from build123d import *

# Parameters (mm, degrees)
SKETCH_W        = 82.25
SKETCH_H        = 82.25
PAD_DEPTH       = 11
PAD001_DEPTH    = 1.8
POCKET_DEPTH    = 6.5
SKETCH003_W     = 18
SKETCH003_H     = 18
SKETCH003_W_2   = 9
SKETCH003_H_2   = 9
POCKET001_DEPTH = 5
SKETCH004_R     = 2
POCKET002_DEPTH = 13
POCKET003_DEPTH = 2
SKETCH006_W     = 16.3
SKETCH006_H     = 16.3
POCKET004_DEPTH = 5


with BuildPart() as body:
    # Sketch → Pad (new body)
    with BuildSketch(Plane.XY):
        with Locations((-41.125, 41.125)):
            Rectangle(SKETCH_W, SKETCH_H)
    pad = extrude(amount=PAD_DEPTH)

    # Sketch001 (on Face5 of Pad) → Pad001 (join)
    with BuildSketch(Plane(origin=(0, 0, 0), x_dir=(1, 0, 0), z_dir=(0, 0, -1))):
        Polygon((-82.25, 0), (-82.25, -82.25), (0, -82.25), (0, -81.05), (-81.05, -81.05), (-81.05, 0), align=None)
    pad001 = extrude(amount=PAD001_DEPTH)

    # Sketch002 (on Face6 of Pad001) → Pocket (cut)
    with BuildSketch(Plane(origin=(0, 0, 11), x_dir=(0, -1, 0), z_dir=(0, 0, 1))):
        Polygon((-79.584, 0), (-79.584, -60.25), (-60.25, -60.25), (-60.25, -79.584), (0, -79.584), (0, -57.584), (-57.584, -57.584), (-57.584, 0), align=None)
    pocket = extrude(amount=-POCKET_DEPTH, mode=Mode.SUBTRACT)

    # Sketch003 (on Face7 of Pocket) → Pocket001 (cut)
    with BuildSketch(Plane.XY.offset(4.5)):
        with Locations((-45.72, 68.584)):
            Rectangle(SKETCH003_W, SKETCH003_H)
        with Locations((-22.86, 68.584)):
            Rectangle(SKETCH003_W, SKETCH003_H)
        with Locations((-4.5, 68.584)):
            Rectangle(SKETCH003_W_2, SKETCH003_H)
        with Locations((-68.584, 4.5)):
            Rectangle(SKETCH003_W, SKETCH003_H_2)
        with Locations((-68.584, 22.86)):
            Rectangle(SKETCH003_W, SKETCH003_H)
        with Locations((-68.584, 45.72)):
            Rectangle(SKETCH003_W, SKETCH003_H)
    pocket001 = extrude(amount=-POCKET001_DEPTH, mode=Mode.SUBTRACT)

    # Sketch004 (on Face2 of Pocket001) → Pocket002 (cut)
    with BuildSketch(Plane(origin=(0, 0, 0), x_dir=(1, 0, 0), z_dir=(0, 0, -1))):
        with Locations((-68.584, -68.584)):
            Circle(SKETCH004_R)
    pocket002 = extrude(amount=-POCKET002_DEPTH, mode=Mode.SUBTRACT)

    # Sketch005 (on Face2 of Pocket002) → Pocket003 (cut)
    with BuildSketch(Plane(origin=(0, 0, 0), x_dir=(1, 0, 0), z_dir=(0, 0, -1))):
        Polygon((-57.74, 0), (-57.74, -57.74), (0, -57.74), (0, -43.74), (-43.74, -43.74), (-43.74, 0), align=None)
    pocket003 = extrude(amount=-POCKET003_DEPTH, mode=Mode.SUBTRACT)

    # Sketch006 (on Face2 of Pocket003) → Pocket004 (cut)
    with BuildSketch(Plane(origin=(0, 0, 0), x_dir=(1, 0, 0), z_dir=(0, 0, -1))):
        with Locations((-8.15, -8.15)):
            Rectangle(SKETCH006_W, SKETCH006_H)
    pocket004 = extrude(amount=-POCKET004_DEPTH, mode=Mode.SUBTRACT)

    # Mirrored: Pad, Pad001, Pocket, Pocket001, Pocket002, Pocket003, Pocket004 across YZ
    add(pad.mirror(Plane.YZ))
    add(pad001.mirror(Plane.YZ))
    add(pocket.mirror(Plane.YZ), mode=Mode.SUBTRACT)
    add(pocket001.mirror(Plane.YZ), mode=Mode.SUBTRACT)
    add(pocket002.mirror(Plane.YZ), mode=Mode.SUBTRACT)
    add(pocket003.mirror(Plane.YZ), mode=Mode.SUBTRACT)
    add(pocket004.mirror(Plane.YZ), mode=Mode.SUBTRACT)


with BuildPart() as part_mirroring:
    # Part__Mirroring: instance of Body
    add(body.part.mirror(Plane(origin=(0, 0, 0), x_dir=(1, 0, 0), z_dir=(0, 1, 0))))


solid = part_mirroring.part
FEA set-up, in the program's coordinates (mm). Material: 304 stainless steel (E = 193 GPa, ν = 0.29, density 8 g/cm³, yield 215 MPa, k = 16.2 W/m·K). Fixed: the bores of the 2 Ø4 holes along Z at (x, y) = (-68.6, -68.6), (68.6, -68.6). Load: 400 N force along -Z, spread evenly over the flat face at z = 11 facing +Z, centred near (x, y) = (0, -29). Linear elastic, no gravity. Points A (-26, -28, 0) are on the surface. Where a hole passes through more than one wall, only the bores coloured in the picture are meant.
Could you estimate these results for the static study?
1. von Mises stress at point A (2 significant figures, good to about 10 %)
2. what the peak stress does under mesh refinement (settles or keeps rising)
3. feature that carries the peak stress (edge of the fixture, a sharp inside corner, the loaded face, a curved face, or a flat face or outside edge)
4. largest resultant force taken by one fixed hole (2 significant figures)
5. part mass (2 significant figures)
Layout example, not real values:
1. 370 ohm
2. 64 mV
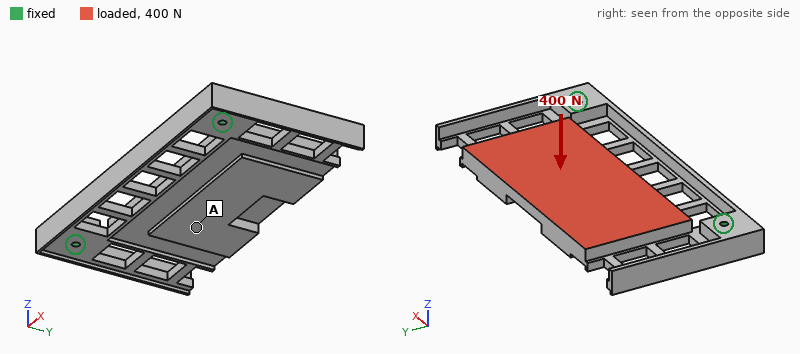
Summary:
1. 7.2 MPa
2. keeps rising
3. a sharp inside corner
4. 240 N
5. 740 g
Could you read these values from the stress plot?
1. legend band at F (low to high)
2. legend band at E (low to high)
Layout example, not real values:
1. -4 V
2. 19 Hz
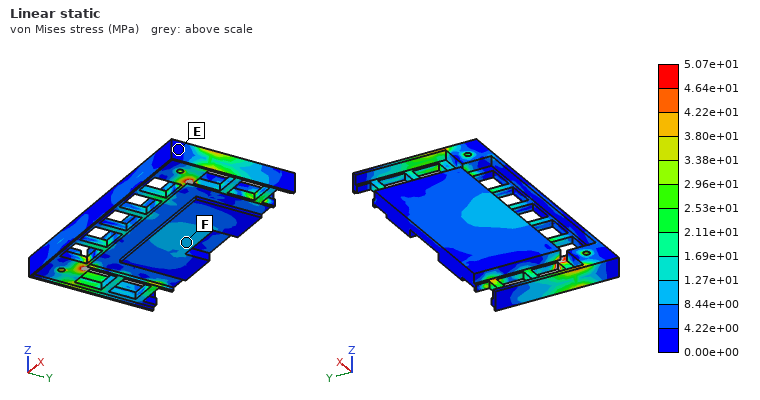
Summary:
1. 8.44e+00 to 1.27e+01 MPa
2. 0.00e+00 to 4.22e+00 MPa
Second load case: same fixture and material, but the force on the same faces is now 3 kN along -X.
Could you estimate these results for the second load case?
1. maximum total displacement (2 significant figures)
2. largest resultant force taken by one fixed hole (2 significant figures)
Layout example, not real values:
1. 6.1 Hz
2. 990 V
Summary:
1. 10 µm
2. 1.7 kN
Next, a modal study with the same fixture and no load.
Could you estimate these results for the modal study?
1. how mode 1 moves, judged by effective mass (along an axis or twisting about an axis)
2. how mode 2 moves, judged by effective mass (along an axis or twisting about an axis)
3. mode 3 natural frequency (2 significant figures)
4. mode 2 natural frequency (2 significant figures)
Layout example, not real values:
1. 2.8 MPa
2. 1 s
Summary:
1. along Z
2. twisting about Y
3. 2400 Hz
4. 1900 Hz
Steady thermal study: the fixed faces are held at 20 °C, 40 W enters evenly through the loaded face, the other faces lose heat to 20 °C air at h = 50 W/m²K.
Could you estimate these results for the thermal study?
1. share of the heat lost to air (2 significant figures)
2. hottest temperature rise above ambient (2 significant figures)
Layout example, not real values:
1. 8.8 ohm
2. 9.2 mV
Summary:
1. 92 %
2. 62 K
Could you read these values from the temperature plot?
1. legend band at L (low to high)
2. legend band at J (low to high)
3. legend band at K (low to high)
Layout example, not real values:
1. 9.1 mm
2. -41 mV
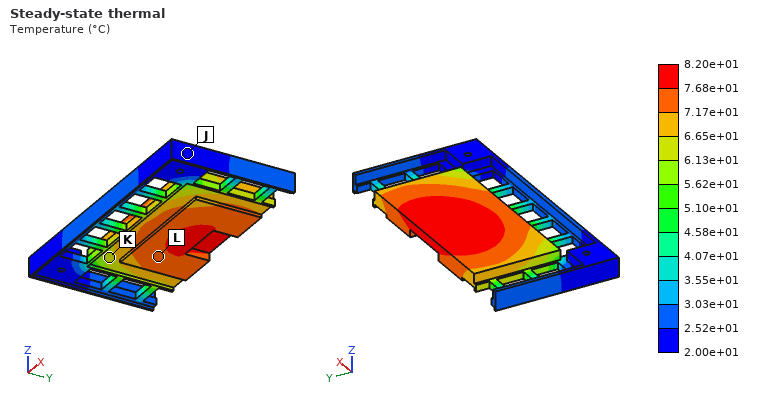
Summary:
1. 7.17e+01 to 7.68e+01 °C
2. 2.00e+01 to 2.52e+01 °C
3. 6.13e+01 to 6.65e+01 °C
